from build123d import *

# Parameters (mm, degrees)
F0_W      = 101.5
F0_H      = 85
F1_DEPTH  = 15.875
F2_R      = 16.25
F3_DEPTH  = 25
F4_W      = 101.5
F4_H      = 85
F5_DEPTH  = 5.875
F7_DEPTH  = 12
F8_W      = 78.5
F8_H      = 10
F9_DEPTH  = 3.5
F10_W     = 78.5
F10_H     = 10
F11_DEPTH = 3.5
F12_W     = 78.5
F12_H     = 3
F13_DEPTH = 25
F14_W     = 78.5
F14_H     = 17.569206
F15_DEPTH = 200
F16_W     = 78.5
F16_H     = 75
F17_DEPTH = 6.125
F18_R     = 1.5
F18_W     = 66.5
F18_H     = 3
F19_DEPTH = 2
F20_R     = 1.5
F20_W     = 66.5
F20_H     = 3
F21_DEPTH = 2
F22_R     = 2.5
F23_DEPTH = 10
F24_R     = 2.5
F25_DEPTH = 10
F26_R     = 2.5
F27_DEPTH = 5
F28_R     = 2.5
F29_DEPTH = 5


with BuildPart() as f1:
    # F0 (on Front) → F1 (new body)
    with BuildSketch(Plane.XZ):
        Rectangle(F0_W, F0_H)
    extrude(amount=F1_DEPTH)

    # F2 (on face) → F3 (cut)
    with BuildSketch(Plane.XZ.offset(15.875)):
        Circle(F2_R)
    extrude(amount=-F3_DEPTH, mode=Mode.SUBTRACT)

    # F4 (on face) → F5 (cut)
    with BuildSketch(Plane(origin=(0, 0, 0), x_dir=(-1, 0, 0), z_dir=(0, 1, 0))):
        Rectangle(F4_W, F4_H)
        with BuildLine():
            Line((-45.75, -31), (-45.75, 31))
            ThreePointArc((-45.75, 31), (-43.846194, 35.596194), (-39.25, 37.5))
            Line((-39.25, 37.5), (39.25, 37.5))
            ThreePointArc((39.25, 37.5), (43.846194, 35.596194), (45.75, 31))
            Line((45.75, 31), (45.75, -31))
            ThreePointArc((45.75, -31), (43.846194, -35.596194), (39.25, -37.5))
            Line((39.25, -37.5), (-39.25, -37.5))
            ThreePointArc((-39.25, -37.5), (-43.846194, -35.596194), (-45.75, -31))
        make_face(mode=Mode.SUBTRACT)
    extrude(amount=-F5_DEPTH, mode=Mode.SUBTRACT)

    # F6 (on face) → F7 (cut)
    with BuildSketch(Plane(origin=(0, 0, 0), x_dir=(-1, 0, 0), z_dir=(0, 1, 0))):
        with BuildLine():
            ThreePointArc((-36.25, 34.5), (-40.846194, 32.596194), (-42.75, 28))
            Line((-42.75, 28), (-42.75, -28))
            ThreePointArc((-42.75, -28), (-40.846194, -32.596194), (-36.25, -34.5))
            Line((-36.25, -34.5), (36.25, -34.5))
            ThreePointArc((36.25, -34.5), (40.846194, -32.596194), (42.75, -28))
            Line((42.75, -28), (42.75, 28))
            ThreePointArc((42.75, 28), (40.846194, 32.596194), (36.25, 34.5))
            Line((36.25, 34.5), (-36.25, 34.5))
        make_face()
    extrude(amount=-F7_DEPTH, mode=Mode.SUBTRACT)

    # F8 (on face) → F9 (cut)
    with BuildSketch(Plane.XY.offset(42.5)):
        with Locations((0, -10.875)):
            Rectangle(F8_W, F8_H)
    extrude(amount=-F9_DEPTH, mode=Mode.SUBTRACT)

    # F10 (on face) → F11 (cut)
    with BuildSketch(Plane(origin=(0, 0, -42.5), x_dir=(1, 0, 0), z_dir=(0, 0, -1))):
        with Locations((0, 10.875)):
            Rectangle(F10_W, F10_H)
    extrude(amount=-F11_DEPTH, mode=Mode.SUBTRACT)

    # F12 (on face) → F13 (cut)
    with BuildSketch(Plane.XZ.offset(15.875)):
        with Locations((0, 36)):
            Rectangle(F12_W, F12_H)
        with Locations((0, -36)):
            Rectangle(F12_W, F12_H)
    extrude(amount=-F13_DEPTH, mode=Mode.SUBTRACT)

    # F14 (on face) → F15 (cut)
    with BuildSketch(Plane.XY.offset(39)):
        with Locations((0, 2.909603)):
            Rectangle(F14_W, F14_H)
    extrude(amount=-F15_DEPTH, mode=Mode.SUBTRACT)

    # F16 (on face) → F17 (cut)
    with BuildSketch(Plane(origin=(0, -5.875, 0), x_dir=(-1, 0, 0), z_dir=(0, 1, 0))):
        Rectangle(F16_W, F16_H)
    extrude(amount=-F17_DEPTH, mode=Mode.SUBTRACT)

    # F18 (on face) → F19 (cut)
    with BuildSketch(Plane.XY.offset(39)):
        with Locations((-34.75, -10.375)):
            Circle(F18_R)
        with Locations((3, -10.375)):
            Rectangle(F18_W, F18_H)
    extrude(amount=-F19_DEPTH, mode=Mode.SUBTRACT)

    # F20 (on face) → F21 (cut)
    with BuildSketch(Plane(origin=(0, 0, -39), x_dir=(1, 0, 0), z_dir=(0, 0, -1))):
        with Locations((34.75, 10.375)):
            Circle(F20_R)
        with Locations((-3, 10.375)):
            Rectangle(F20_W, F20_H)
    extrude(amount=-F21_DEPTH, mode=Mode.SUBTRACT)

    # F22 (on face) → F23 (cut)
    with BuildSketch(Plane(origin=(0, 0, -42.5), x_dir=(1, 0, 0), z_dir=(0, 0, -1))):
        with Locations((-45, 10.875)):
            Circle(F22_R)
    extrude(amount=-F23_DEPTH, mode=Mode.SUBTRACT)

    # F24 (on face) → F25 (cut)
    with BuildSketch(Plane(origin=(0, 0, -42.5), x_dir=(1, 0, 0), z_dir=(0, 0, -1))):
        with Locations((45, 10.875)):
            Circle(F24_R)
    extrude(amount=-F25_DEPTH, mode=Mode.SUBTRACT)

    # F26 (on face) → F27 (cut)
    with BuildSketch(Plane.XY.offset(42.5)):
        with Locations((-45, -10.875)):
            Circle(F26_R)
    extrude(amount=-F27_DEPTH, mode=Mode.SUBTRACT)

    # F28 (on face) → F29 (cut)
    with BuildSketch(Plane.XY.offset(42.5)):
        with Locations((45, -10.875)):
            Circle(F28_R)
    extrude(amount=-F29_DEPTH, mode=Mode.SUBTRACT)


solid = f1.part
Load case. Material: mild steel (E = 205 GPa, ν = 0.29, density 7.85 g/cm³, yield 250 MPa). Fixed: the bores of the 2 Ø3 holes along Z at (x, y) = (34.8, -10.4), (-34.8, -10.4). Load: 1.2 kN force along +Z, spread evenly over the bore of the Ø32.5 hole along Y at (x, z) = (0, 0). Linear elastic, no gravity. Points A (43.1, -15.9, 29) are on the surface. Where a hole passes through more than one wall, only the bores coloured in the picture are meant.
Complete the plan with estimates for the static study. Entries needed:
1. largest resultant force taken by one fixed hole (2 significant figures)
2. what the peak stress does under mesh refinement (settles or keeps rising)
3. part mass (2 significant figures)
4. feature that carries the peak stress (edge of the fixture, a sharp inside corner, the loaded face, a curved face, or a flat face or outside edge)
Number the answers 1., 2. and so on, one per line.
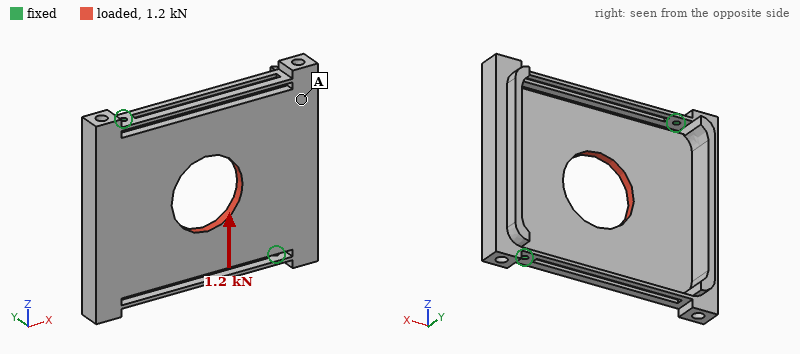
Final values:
1. 600 N
2. keeps rising
3. 300 g
4. edge of the fixture
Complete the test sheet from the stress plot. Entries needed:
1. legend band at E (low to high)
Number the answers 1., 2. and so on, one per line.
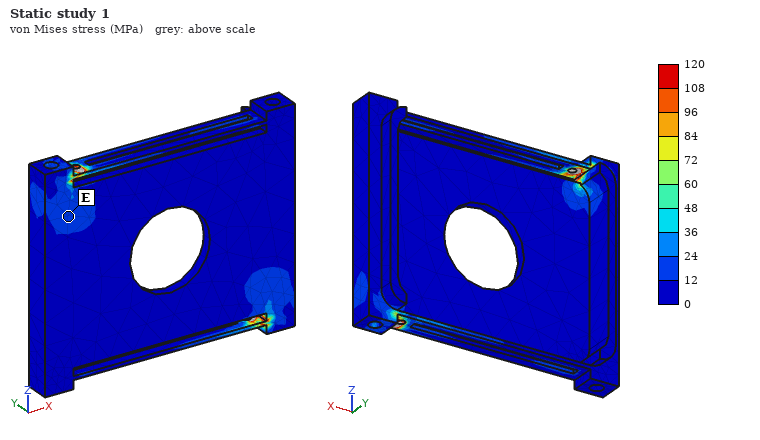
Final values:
1. 12 to 24 MPa
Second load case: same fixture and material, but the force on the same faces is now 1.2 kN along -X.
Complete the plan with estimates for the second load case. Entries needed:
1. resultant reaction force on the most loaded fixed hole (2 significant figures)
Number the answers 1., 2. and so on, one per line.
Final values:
1. 600 N
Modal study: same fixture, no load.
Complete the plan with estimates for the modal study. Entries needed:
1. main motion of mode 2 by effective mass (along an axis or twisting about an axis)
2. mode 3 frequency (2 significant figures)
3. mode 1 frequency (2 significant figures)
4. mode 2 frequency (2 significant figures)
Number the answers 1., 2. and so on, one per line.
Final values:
1. along Y
2. 1500 Hz
3. 390 Hz
4. 590 Hz
